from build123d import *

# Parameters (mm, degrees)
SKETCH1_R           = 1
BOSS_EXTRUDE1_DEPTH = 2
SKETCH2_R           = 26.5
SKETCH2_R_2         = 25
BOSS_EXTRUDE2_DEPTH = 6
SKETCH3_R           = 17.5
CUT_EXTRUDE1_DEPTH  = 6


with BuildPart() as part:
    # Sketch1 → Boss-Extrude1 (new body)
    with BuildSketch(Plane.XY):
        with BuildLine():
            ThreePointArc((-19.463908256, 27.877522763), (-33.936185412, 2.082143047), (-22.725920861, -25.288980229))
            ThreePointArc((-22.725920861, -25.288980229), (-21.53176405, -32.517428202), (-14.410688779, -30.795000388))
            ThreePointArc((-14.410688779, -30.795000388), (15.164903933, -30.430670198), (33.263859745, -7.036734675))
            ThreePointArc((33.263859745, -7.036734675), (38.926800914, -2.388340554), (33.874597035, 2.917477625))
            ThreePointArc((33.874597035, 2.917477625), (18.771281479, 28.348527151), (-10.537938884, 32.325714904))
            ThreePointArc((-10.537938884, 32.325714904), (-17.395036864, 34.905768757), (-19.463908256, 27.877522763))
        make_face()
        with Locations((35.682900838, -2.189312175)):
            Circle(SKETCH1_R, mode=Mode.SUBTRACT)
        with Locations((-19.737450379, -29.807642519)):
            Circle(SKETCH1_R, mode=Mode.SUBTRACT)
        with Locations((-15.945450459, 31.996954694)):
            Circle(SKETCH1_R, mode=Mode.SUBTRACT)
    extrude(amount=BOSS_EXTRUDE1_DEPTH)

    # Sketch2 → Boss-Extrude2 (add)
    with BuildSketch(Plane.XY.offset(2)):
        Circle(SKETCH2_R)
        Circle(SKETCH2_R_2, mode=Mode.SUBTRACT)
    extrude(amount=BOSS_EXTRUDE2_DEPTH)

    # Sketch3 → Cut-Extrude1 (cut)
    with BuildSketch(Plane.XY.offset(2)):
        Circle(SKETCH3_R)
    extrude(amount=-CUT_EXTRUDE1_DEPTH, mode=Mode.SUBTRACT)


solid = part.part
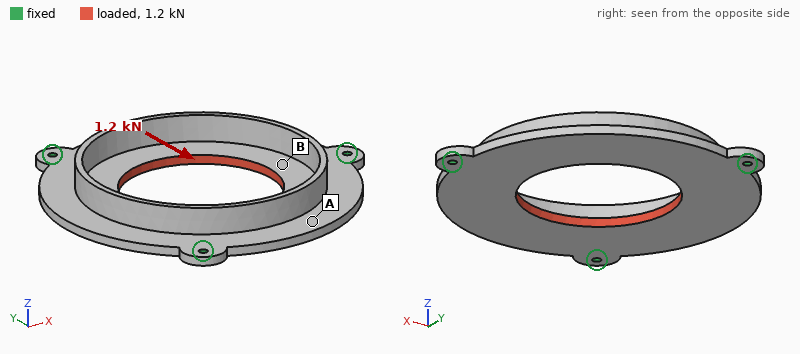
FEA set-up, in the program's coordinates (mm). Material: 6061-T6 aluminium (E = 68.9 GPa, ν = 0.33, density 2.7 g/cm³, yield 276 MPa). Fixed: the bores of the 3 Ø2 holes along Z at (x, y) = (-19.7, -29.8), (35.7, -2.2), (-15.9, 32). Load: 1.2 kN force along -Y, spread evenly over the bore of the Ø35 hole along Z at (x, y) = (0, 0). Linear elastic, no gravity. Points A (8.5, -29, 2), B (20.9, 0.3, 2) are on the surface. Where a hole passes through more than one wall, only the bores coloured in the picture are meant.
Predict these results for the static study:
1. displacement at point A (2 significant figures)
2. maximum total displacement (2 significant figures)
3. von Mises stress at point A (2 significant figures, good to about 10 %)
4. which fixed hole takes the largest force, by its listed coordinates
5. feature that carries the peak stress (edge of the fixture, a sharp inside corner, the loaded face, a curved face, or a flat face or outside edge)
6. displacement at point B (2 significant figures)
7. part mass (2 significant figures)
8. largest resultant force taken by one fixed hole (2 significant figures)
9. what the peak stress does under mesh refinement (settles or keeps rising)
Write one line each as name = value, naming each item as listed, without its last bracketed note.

displacement at point A = 13 µm
maximum total displacement = 16 µm
von Mises stress at point A = 9.7 MPa
which fixed hole takes the largest force, by its listed coordinates = (35.7, -2.2)
feature that carries the peak stress = edge of the fixture
displacement at point B = 13 µm
part mass = 19 g
largest resultant force taken by one fixed hole = 450 N
what the peak stress does under mesh refinement = keeps rising
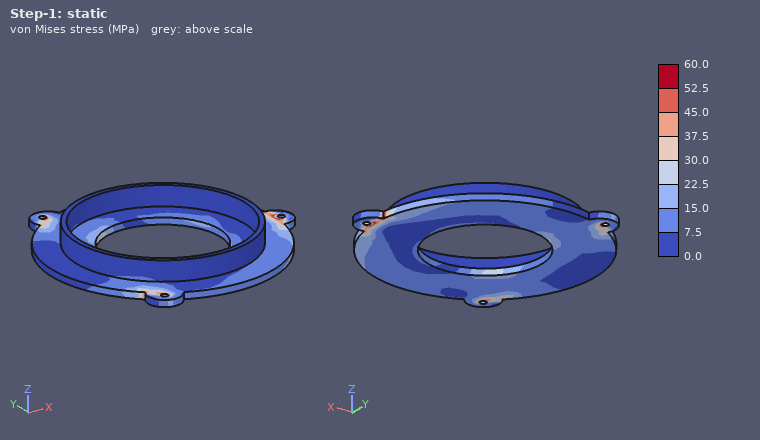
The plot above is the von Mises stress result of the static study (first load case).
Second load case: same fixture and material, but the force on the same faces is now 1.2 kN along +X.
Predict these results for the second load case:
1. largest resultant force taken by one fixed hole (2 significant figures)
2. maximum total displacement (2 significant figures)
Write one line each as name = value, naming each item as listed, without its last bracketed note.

largest resultant force taken by one fixed hole = 430 N
maximum total displacement = 18 µm
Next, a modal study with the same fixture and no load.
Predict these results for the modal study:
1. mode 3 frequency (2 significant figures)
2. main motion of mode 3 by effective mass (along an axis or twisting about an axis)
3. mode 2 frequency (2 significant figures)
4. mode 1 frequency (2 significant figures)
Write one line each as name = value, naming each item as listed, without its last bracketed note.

mode 3 frequency = 3200 Hz
main motion of mode 3 by effective mass = along Z
mode 2 frequency = 2600 Hz
mode 1 frequency = 2600 Hz
